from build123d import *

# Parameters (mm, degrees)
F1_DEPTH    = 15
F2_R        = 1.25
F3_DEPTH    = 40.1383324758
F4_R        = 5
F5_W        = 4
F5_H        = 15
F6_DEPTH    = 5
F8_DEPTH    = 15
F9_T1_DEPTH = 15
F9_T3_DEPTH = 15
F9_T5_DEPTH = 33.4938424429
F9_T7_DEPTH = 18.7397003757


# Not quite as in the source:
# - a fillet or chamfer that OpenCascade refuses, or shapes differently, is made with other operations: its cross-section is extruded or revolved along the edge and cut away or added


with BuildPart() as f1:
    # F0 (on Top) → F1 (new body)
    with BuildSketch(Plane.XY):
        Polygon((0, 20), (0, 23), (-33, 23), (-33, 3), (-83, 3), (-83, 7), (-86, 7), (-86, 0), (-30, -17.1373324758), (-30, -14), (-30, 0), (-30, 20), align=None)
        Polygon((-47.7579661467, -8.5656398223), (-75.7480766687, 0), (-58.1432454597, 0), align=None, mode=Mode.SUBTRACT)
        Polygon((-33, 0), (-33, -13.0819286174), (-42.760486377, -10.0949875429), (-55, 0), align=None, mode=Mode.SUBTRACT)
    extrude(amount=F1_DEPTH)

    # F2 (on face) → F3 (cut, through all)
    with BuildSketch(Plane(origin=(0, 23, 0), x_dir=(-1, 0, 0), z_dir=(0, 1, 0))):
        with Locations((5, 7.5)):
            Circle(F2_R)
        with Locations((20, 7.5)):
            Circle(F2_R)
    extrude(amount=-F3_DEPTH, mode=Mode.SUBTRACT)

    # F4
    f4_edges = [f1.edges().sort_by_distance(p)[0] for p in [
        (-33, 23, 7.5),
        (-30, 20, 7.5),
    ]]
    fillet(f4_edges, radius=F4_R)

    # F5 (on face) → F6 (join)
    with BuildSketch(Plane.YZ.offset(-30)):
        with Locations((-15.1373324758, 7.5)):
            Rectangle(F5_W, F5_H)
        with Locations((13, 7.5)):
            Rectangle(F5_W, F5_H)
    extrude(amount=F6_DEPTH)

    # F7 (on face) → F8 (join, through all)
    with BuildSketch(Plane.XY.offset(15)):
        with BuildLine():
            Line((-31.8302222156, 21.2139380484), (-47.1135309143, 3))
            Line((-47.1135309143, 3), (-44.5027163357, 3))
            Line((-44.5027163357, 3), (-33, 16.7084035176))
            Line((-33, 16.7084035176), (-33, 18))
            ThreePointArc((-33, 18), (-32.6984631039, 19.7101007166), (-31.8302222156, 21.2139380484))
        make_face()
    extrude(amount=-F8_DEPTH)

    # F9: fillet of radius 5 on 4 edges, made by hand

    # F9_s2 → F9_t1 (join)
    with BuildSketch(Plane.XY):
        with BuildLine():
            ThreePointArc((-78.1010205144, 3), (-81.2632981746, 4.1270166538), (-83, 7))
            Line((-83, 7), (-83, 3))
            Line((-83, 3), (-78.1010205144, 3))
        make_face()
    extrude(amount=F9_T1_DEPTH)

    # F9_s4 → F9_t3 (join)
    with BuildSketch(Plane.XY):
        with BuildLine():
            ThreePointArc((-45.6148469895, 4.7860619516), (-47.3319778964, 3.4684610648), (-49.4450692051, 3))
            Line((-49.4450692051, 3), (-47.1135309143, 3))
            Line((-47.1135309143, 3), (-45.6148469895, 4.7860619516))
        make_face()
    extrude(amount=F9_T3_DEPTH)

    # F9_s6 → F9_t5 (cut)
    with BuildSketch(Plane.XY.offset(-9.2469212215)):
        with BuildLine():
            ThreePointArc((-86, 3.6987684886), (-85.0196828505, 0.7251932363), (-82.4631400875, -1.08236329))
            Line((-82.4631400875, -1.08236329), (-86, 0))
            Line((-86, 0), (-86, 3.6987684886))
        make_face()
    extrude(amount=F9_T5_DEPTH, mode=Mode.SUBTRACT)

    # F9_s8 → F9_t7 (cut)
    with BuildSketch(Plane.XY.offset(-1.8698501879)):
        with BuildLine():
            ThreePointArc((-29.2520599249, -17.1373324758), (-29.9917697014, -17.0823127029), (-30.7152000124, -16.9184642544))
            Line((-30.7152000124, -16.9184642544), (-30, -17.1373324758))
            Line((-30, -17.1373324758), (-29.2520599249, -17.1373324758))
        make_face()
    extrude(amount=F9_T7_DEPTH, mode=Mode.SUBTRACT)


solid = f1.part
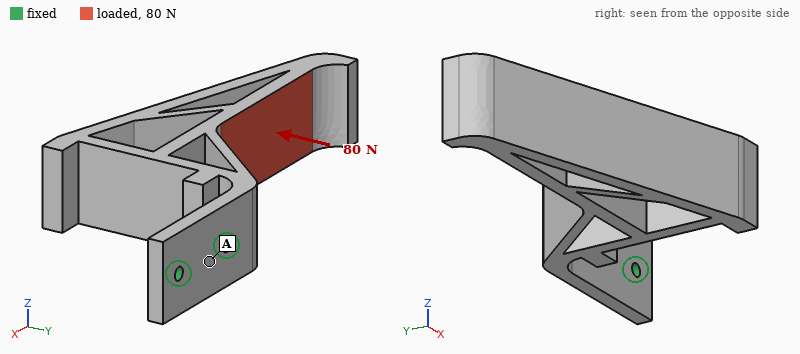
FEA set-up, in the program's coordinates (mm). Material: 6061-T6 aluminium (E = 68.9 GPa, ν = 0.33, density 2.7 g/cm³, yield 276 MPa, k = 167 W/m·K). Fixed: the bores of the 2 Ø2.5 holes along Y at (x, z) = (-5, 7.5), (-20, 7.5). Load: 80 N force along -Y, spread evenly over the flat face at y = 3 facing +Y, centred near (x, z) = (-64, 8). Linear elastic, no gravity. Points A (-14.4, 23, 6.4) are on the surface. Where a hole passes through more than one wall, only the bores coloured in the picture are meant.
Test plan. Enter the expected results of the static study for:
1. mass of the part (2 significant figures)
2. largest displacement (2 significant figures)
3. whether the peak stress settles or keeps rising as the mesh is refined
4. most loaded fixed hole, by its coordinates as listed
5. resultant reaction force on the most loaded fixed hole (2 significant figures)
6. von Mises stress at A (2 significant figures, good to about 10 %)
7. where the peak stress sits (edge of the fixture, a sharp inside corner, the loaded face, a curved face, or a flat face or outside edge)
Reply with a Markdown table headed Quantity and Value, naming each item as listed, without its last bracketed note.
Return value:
| Quantity | Value |
|---|---|
| mass of the part | 26 g |
| largest displacement | 0.99 mm |
| whether the peak stress settles or keeps rising as the mesh is refined | keeps rising |
| most loaded fixed hole, by its coordinates as listed | (-20, 7.5) |
| resultant reaction force on the most loaded fixed hole | 150 N |
| von Mises stress at A | 22 MPa |
| where the peak stress sits | edge of the fixture |
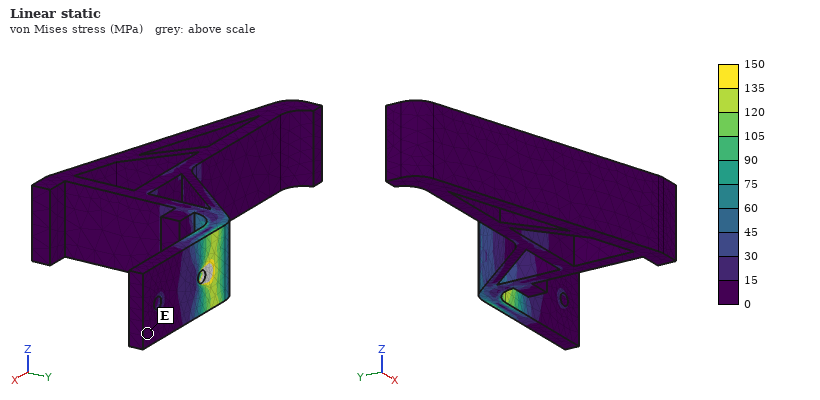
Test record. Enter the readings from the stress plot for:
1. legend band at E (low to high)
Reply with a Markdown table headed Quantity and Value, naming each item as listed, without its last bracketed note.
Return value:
| Quantity | Value |
|---|---|
| legend band at E | 0 to 15 MPa |
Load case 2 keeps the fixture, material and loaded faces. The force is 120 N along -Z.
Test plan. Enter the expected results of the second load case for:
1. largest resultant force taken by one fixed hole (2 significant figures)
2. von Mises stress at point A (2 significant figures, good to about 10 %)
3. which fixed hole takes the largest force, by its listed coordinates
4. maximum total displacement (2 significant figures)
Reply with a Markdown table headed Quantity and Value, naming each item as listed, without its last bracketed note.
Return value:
| Quantity | Value |
|---|---|
| largest resultant force taken by one fixed hole | 390 N |
| von Mises stress at point A | 23 MPa |
| which fixed hole takes the largest force, by its listed coordinates | (-20, 7.5) |
| maximum total displacement | 0.29 mm |
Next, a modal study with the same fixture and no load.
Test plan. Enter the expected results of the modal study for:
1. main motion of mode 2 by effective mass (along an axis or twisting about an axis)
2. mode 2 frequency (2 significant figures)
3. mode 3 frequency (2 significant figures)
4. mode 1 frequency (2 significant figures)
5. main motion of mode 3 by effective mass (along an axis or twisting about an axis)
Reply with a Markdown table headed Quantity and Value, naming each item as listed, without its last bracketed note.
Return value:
| Quantity | Value |
|---|---|
| main motion of mode 2 by effective mass | along Z |
| mode 2 frequency | 850 Hz |
| mode 3 frequency | 1800 Hz |
| mode 1 frequency | 400 Hz |
| main motion of mode 3 by effective mass | twisting about Y |
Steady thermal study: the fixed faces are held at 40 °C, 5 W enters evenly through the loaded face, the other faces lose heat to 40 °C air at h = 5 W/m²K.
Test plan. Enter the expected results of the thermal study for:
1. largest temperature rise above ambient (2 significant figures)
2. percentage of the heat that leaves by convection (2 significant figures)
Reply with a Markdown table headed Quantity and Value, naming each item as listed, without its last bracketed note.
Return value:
| Quantity | Value |
|---|---|
| largest temperature rise above ambient | 22 K |
| percentage of the heat that leaves by convection | 9.7 % |
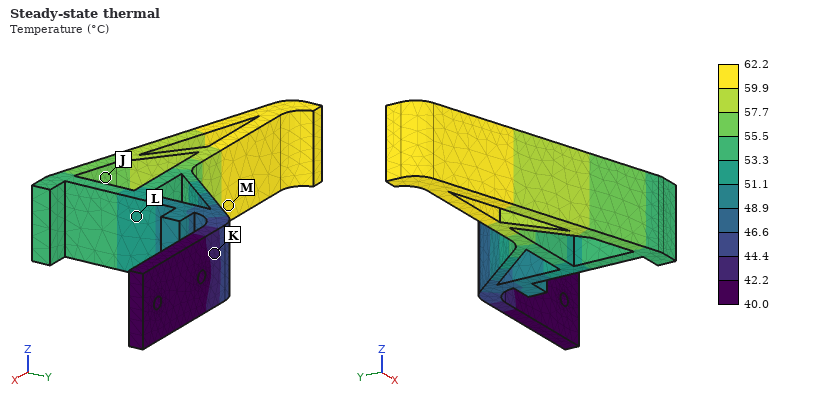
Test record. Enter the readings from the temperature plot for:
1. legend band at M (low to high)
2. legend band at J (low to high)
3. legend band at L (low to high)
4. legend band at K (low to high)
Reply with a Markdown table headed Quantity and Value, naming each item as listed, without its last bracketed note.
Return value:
| Quantity | Value |
|---|---|
| legend band at M | 59.9 to 62.2 °C |
| legend band at J | 55.5 to 57.7 °C |
| legend band at L | 51.1 to 53.3 °C |
| legend band at K | 42.2 to 44.4 °C |
